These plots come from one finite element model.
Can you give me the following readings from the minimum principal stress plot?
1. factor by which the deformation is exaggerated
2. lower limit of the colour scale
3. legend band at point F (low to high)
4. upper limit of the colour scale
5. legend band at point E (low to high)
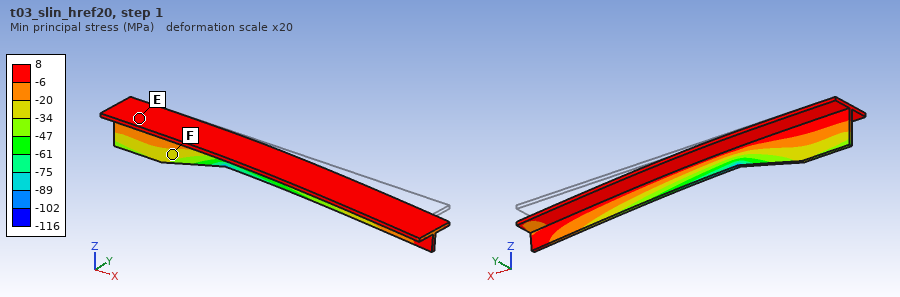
20
-116 MPa
-34 to -20 MPa
8 MPa
-6 to 8 MPa
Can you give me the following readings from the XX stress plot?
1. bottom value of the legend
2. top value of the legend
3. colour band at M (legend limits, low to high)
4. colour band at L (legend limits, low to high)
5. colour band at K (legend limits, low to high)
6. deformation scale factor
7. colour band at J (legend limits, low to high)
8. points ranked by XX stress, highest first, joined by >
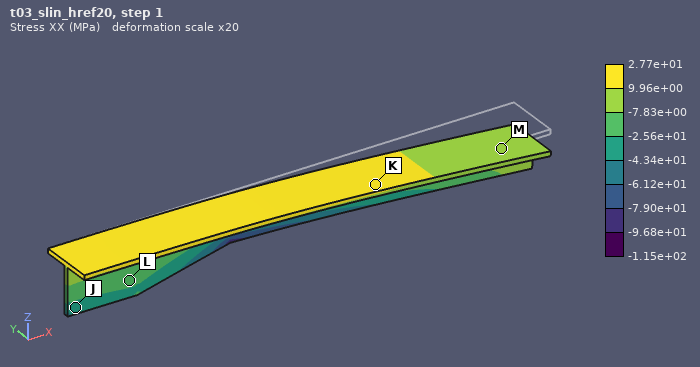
-1.15e+02 MPa
2.77e+01 MPa
-7.83e+00 to 9.96e+00 MPa
-2.56e+01 to -7.83e+00 MPa
9.96e+00 to 2.77e+01 MPa
20
-4.34e+01 to -2.56e+01 MPa
K > M > L > J
